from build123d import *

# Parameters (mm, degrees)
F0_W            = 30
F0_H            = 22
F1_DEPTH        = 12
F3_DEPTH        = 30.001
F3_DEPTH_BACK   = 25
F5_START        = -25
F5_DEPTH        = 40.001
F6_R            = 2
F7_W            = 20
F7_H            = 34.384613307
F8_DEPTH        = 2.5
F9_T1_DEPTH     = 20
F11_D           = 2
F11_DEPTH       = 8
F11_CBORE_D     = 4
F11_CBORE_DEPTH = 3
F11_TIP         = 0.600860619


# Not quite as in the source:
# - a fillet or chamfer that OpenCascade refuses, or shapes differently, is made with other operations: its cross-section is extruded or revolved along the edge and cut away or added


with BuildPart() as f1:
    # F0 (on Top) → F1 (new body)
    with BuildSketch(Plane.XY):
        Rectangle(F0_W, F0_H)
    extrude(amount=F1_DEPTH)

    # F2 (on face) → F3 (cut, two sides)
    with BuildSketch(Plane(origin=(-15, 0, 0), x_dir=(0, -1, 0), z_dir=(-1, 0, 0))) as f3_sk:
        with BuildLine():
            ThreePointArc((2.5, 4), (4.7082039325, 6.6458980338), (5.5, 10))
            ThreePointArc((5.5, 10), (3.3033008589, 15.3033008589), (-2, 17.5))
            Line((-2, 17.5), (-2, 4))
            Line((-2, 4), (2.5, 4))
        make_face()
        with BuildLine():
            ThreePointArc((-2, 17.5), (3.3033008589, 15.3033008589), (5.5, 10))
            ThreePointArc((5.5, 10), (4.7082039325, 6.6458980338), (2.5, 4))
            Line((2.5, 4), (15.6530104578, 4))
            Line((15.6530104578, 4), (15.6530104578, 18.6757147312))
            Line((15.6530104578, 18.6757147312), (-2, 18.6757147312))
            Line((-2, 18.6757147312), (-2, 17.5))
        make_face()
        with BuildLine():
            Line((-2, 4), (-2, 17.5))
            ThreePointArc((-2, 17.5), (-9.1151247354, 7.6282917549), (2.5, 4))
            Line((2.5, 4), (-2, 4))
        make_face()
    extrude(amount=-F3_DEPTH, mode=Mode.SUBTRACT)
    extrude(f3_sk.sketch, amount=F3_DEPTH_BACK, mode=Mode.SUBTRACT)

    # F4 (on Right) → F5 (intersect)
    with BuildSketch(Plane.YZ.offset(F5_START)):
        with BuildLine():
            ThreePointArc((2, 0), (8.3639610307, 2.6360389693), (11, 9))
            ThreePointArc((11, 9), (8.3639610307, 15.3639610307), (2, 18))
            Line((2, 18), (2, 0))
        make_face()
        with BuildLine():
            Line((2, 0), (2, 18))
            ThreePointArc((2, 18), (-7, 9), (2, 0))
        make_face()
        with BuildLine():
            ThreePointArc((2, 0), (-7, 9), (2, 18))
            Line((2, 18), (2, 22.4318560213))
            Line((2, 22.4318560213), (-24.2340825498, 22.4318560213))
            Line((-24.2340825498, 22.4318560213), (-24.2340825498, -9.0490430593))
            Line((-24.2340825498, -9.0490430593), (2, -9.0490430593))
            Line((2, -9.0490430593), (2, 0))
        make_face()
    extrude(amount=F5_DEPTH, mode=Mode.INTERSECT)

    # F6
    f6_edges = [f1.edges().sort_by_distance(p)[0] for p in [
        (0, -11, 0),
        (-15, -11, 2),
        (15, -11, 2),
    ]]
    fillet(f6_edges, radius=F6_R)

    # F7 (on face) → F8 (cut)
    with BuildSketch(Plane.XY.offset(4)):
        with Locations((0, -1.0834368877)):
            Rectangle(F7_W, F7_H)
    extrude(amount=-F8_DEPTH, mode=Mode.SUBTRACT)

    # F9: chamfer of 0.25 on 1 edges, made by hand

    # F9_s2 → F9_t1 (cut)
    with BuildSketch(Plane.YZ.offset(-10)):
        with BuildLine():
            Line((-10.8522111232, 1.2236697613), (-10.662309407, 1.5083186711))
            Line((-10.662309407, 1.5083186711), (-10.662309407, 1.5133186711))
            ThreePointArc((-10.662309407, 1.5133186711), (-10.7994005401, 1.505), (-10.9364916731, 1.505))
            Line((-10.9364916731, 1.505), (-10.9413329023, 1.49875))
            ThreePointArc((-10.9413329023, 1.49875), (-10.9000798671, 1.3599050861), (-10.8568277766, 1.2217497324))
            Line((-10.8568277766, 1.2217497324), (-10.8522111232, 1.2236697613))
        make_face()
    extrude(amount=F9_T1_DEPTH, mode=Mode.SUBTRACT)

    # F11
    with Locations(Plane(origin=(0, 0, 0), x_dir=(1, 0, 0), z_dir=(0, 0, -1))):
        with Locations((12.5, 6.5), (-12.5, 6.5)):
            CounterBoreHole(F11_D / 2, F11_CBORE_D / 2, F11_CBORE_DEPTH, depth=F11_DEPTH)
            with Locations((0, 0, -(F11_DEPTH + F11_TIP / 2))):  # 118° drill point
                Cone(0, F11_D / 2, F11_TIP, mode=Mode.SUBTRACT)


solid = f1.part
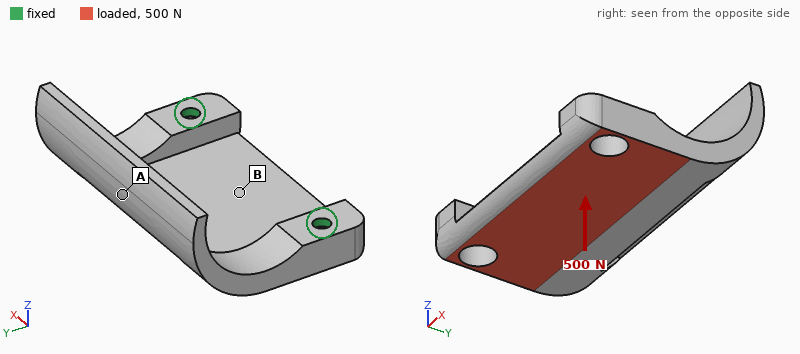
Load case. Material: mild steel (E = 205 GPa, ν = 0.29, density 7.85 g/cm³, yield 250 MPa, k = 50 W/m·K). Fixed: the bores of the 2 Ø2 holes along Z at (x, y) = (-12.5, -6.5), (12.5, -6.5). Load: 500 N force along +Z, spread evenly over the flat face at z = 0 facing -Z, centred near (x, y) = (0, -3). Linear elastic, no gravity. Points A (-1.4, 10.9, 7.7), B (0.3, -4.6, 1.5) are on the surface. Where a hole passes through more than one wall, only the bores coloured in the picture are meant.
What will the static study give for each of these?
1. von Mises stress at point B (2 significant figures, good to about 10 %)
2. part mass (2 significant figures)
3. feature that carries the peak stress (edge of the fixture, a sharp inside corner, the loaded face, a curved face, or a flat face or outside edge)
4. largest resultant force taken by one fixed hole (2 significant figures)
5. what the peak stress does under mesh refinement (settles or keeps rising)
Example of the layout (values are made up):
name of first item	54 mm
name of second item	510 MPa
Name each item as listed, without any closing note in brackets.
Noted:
von Mises stress at point B	58 MPa
part mass	11 g
feature that carries the peak stress	edge of the fixture
largest resultant force taken by one fixed hole	320 N
what the peak stress does under mesh refinement	keeps rising
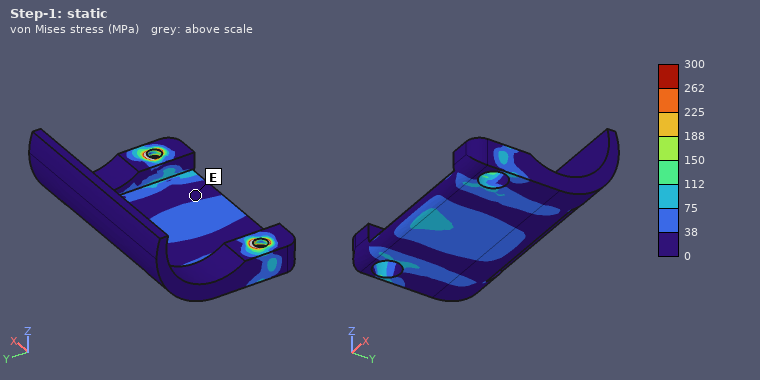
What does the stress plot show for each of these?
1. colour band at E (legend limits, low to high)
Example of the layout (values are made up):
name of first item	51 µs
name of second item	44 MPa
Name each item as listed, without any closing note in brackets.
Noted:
colour band at E	0 to 38 MPa
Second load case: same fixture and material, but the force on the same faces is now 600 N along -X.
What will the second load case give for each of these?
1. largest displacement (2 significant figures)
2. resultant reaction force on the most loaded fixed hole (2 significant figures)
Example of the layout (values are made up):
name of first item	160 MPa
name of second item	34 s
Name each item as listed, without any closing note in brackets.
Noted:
largest displacement	5.9 µm
resultant reaction force on the most loaded fixed hole	310 N
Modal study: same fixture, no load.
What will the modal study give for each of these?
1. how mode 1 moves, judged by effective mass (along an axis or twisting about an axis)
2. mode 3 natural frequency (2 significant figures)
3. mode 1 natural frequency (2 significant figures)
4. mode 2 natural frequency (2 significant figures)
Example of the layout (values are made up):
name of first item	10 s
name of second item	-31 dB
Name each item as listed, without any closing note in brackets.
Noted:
how mode 1 moves, judged by effective mass	along Z
mode 3 natural frequency	8200 Hz
mode 1 natural frequency	2900 Hz
mode 2 natural frequency	5400 Hz
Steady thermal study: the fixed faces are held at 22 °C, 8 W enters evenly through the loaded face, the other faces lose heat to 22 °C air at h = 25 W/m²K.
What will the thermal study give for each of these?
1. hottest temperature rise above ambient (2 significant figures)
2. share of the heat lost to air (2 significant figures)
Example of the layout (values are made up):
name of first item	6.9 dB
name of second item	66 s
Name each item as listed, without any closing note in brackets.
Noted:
hottest temperature rise above ambient	35 K
share of the heat lost to air	12 %
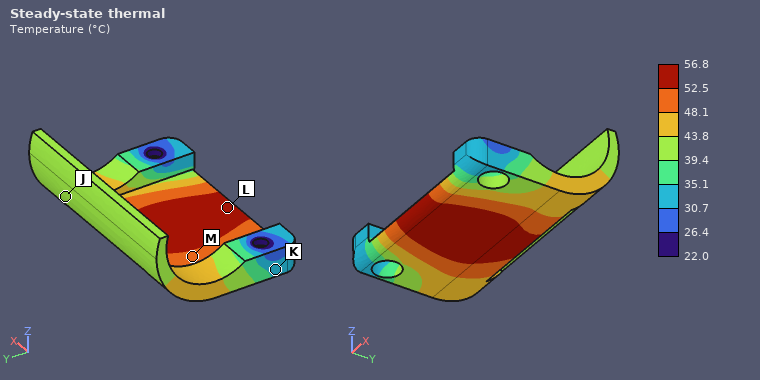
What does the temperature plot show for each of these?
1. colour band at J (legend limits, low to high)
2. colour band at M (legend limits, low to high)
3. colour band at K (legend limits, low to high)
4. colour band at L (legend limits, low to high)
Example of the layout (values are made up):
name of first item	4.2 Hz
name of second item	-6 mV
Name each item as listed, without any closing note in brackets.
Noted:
colour band at J	39.4 to 43.8 °C
colour band at M	48.1 to 52.5 °C
colour band at K	30.7 to 35.1 °C
colour band at L	52.5 to 56.8 °C
